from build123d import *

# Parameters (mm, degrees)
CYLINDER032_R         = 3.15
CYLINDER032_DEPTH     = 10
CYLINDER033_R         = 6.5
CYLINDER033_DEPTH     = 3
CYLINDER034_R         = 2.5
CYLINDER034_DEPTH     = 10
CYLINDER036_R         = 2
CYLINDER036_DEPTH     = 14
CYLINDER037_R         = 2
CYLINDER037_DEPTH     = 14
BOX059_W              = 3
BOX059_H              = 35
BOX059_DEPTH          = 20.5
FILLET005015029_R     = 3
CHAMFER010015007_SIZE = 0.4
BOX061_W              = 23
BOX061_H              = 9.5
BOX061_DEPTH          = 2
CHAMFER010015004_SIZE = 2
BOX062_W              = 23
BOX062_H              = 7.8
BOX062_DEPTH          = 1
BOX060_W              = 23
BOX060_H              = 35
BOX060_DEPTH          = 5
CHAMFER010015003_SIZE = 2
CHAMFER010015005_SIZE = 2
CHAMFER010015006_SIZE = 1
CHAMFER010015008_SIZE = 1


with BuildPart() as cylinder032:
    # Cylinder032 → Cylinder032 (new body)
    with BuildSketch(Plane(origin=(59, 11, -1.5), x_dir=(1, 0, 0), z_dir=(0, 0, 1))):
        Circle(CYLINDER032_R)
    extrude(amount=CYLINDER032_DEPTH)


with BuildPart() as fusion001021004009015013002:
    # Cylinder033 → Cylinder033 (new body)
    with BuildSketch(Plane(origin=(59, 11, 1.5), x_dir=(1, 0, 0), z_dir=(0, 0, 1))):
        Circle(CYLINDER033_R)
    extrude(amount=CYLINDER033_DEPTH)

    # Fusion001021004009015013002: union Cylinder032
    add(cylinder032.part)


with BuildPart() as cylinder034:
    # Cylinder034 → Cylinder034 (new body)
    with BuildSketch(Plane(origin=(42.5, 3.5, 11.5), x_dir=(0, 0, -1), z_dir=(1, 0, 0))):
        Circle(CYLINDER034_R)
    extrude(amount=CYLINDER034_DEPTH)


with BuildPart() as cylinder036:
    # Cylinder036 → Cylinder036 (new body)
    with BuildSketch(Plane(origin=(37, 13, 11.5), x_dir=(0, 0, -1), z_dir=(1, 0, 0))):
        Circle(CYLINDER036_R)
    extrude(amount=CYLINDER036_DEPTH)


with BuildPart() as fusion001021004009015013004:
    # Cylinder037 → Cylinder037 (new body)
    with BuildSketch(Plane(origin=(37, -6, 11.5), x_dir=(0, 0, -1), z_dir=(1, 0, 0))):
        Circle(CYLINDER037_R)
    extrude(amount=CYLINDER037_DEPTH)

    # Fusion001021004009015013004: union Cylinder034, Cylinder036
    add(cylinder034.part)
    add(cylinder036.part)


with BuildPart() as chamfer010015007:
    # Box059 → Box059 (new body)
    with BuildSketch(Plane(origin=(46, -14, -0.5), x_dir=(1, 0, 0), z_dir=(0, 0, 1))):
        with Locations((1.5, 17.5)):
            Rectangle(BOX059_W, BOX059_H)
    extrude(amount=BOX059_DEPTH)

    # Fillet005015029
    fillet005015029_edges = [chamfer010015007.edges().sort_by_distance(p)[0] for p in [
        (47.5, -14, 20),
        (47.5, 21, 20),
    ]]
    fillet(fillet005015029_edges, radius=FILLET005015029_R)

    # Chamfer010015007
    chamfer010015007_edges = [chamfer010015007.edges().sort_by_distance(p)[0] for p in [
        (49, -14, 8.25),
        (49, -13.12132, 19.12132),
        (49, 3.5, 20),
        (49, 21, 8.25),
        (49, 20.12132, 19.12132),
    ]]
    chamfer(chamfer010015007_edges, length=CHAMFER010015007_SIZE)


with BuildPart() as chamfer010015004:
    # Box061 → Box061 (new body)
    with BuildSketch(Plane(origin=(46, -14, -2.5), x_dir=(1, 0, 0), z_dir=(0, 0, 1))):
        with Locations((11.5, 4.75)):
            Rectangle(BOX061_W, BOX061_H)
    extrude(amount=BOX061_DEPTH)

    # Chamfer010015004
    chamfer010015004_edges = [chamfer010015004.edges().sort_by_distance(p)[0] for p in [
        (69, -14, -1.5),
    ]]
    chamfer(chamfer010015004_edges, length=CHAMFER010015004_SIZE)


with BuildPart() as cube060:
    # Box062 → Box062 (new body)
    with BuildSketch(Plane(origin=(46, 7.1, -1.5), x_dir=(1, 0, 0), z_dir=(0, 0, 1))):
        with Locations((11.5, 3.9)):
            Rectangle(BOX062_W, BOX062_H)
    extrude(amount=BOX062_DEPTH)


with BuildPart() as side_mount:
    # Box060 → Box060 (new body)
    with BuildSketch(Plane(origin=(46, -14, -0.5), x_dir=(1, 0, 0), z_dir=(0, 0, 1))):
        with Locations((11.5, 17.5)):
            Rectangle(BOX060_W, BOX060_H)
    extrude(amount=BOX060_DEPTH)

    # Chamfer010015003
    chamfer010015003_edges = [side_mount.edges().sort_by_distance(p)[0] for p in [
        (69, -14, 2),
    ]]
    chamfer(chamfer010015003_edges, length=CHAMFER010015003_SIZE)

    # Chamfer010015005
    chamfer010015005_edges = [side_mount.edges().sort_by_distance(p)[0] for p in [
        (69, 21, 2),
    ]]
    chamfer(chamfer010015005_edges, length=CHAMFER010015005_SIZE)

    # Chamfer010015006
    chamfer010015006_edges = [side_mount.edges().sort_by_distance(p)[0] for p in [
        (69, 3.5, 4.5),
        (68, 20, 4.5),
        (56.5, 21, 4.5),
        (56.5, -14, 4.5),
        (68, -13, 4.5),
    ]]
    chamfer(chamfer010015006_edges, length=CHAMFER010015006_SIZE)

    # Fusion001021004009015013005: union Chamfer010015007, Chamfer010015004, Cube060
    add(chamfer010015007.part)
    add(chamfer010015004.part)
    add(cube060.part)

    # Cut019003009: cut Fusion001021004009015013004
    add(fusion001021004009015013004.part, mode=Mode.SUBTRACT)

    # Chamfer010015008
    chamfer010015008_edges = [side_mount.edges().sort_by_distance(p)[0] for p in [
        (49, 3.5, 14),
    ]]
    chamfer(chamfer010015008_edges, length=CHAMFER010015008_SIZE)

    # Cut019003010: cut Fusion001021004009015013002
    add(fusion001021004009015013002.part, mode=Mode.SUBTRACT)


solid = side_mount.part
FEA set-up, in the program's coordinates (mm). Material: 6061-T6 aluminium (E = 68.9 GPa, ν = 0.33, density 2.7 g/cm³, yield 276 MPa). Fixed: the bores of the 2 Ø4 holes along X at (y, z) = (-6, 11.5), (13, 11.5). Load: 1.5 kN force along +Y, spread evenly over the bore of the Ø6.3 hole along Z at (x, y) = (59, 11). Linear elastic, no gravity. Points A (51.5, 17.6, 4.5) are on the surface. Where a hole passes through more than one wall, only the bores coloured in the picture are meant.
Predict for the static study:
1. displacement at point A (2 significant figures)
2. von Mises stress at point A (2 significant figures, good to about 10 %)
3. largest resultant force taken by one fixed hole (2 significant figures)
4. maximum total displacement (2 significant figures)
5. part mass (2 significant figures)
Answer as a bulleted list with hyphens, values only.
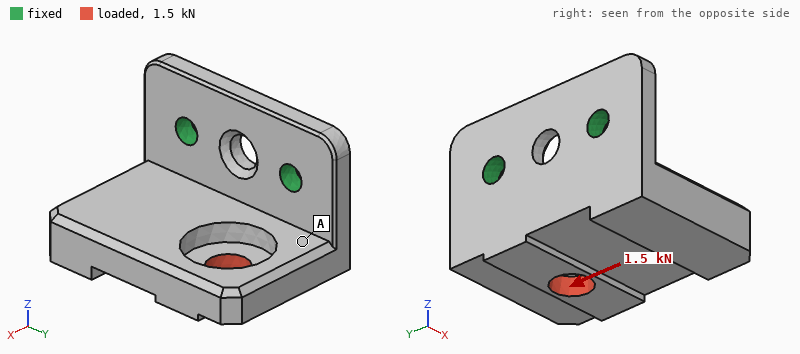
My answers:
- 38 µm
- 37 MPa
- 1.3 kN
- 85 µm
- 15 g
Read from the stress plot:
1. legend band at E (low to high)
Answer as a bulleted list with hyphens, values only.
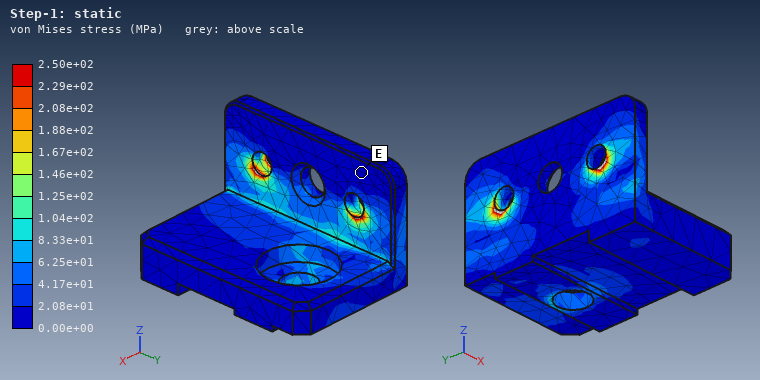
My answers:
- 0.00e+00 to 2.08e+01 MPa
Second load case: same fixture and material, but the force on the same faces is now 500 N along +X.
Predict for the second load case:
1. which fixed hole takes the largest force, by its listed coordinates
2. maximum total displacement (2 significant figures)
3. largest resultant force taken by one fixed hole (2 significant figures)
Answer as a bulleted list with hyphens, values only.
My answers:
- (13, 11.5)
- 0.14 mm
- 420 N
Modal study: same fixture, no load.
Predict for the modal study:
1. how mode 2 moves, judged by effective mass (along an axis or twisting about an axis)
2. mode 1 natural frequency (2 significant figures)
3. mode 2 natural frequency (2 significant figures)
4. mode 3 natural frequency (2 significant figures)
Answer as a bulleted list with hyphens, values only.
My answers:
- along Y
- 2800 Hz
- 6600 Hz
- 11 kHz
